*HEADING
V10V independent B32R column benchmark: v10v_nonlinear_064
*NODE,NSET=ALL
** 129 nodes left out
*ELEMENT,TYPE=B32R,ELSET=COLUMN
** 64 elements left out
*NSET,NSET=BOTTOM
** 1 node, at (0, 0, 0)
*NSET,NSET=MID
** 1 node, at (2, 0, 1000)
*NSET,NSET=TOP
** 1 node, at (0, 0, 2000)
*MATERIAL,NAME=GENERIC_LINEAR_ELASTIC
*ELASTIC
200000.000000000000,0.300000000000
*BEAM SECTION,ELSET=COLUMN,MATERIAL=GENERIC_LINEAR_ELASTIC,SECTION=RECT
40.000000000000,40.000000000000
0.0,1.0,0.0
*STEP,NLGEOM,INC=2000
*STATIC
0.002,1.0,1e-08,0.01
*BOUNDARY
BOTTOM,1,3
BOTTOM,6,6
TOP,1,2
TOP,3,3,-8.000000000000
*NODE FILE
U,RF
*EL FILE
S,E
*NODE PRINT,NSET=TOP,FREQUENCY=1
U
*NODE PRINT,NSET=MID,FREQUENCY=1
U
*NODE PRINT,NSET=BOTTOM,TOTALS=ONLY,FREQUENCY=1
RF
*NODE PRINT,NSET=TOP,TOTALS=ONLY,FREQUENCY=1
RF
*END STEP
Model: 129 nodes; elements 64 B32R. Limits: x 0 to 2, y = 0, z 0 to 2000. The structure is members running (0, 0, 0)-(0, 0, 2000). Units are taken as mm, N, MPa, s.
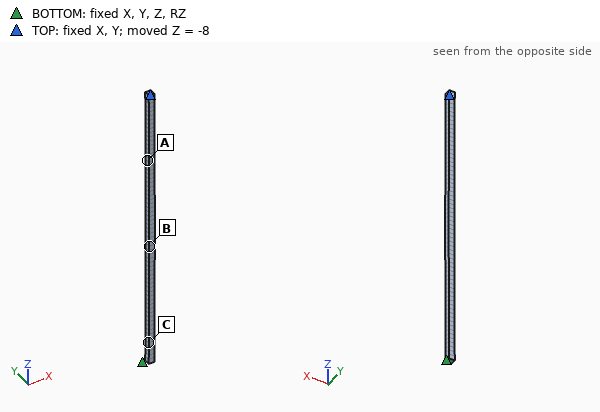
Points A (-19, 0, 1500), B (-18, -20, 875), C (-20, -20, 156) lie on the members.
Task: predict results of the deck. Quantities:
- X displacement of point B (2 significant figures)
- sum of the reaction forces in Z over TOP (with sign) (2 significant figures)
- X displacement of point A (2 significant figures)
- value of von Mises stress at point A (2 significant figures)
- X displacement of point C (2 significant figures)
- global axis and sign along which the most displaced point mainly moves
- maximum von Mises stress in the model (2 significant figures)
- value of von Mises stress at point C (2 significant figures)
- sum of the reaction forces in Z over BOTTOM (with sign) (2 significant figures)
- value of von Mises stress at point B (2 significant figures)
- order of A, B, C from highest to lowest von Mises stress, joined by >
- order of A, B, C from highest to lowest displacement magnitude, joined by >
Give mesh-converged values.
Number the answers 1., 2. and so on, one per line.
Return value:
1. 74 mm
2. -1.0e+05 N
3. 53 mm
4. 590 MPa
5. 18 mm
6. +X
7. 800 MPa
8. 240 MPa
9. 1.0e+05 N
10. 790 MPa
11. B > A > C
12. B > A > C
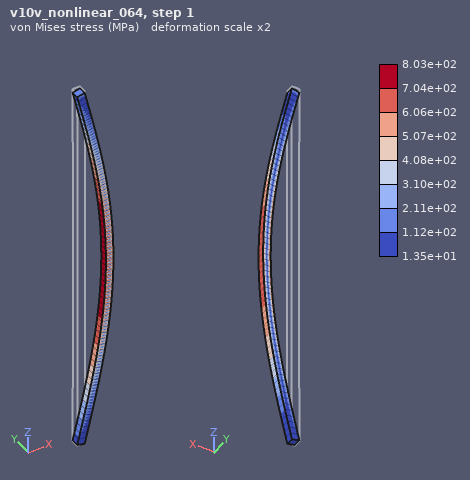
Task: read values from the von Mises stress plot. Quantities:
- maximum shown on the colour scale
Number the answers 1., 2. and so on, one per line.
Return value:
1. 8.03e+02 MPa
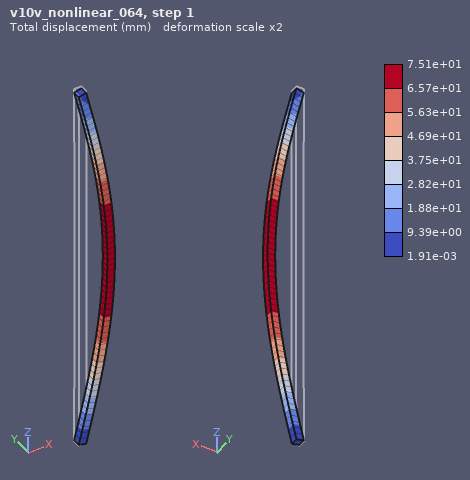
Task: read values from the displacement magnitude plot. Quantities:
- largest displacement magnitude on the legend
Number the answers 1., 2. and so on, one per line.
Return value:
1. 7.51e+01 mm
